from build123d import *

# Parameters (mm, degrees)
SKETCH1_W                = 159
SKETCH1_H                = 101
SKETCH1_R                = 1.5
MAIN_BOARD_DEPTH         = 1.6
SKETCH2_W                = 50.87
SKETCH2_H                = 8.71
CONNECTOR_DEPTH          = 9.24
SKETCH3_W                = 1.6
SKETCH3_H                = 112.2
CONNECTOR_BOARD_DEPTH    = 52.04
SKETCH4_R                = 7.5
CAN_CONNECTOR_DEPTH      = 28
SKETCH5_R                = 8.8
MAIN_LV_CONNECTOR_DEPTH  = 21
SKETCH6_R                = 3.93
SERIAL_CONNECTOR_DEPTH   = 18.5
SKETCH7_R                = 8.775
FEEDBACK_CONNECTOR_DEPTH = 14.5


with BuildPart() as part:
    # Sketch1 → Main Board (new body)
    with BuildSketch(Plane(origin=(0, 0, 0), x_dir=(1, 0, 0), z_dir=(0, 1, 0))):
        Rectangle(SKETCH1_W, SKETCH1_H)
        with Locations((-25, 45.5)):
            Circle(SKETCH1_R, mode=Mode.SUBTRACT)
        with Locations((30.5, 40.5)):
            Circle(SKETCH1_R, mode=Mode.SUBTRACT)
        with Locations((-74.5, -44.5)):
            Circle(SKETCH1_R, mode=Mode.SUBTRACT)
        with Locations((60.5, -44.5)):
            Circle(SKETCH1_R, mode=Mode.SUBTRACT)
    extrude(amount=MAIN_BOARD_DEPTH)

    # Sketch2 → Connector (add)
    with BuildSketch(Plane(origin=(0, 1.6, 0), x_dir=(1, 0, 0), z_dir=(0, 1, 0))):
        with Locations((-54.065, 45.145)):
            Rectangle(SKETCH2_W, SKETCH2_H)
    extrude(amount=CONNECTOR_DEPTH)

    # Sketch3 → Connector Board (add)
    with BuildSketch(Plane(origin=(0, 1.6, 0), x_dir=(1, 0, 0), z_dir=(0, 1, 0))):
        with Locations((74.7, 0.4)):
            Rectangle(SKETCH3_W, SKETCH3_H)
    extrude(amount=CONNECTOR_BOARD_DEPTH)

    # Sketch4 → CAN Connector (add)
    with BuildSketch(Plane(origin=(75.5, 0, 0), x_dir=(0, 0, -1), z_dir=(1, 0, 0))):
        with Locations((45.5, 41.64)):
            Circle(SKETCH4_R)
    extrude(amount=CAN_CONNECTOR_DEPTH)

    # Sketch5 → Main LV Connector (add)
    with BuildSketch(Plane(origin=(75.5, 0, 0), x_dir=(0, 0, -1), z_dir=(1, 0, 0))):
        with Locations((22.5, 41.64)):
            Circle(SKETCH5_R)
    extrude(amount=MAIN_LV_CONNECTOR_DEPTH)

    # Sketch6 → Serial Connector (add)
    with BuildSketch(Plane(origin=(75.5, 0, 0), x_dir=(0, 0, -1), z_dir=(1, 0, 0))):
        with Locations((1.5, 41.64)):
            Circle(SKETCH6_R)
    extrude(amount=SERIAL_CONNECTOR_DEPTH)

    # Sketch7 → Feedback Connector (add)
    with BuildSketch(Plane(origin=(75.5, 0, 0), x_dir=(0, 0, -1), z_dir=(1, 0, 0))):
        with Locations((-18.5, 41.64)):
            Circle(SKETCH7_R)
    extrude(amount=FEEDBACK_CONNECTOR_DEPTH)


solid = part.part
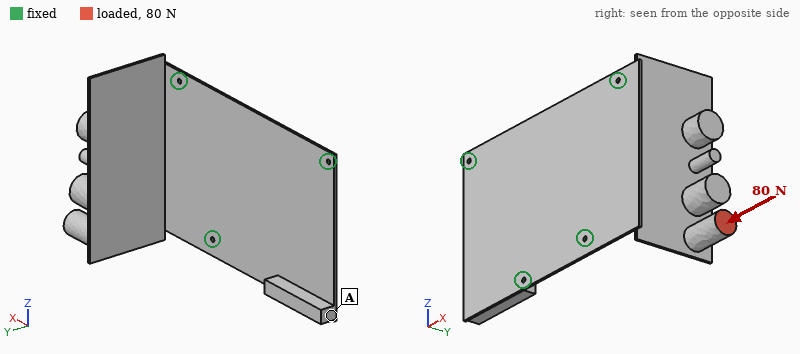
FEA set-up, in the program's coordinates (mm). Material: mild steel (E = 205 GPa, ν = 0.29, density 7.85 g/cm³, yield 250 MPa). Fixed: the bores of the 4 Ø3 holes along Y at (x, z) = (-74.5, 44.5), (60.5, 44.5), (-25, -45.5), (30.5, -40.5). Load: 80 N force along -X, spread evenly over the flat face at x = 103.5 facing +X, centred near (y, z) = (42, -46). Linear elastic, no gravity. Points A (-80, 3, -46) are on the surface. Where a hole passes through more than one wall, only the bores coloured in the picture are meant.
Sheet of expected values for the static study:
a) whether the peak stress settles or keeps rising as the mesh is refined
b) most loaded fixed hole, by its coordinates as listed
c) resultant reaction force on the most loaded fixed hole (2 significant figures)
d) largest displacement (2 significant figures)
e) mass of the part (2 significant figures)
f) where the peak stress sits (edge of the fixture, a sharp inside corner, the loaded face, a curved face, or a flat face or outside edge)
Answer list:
keeps rising
(30.5, -40.5)
66 N
1.8 mm
420 g
edge of the fixture
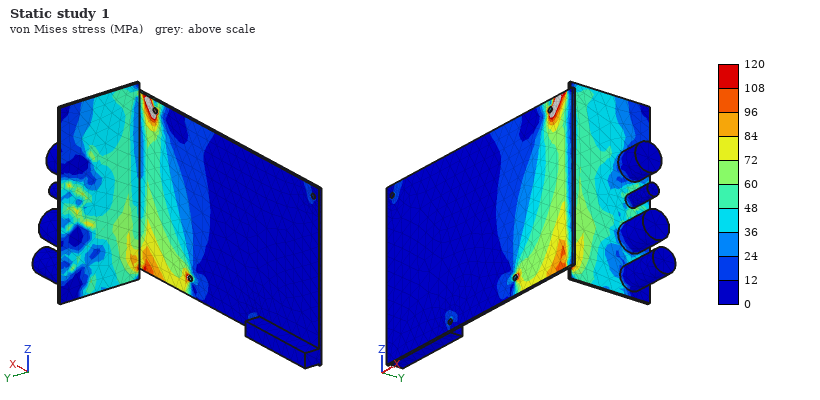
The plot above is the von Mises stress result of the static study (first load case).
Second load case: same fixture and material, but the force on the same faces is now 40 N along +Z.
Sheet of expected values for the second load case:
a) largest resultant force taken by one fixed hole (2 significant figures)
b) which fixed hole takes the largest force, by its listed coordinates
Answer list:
41 N
(60.5, 44.5)
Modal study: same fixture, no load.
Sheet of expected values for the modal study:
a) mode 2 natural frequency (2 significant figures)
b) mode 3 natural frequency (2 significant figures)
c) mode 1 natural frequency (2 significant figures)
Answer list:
260 Hz
370 Hz
100 Hz
